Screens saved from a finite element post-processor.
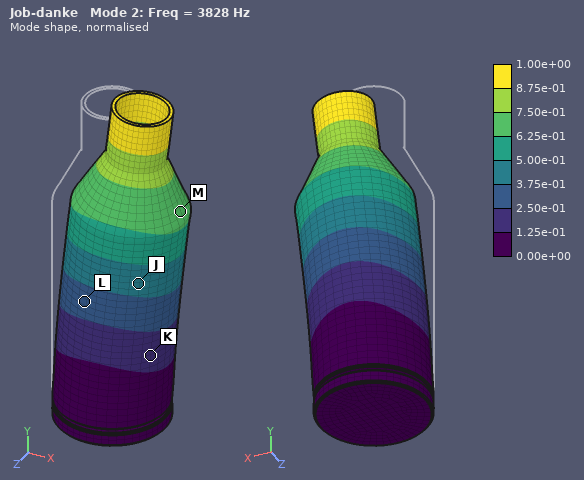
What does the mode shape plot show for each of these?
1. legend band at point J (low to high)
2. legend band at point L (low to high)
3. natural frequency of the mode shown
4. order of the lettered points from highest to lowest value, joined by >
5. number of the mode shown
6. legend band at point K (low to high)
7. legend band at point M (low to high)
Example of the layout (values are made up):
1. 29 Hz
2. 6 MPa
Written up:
1. 3.75e-01 to 5.00e-01
2. 2.50e-01 to 3.75e-01
3. 3828 Hz
4. M > J > L > K
5. 2
6. 1.25e-01 to 2.50e-01
7. 6.25e-01 to 7.50e-01
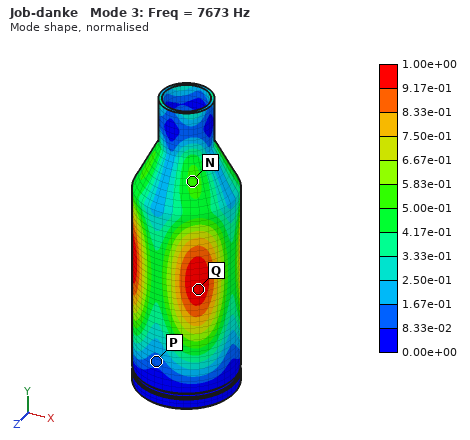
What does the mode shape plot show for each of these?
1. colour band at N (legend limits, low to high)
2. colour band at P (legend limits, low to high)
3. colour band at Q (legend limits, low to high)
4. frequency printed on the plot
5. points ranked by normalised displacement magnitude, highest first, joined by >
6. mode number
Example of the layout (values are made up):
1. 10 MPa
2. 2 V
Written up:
1. 5.00e-01 to 5.83e-01
2. 8.33e-02 to 1.67e-01
3. 9.17e-01 to 1.00e+00
4. 7673 Hz
5. Q > N > P
6. 3
